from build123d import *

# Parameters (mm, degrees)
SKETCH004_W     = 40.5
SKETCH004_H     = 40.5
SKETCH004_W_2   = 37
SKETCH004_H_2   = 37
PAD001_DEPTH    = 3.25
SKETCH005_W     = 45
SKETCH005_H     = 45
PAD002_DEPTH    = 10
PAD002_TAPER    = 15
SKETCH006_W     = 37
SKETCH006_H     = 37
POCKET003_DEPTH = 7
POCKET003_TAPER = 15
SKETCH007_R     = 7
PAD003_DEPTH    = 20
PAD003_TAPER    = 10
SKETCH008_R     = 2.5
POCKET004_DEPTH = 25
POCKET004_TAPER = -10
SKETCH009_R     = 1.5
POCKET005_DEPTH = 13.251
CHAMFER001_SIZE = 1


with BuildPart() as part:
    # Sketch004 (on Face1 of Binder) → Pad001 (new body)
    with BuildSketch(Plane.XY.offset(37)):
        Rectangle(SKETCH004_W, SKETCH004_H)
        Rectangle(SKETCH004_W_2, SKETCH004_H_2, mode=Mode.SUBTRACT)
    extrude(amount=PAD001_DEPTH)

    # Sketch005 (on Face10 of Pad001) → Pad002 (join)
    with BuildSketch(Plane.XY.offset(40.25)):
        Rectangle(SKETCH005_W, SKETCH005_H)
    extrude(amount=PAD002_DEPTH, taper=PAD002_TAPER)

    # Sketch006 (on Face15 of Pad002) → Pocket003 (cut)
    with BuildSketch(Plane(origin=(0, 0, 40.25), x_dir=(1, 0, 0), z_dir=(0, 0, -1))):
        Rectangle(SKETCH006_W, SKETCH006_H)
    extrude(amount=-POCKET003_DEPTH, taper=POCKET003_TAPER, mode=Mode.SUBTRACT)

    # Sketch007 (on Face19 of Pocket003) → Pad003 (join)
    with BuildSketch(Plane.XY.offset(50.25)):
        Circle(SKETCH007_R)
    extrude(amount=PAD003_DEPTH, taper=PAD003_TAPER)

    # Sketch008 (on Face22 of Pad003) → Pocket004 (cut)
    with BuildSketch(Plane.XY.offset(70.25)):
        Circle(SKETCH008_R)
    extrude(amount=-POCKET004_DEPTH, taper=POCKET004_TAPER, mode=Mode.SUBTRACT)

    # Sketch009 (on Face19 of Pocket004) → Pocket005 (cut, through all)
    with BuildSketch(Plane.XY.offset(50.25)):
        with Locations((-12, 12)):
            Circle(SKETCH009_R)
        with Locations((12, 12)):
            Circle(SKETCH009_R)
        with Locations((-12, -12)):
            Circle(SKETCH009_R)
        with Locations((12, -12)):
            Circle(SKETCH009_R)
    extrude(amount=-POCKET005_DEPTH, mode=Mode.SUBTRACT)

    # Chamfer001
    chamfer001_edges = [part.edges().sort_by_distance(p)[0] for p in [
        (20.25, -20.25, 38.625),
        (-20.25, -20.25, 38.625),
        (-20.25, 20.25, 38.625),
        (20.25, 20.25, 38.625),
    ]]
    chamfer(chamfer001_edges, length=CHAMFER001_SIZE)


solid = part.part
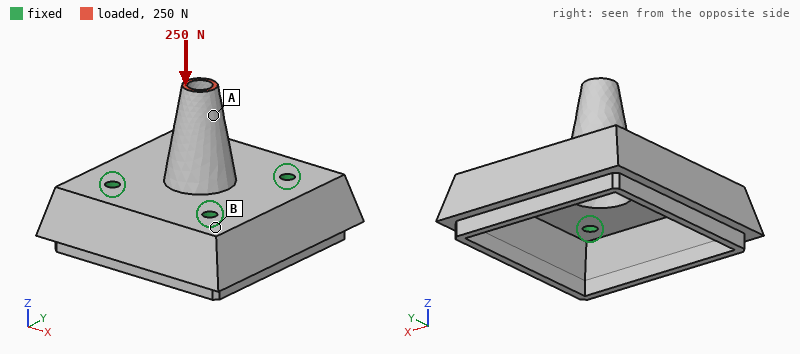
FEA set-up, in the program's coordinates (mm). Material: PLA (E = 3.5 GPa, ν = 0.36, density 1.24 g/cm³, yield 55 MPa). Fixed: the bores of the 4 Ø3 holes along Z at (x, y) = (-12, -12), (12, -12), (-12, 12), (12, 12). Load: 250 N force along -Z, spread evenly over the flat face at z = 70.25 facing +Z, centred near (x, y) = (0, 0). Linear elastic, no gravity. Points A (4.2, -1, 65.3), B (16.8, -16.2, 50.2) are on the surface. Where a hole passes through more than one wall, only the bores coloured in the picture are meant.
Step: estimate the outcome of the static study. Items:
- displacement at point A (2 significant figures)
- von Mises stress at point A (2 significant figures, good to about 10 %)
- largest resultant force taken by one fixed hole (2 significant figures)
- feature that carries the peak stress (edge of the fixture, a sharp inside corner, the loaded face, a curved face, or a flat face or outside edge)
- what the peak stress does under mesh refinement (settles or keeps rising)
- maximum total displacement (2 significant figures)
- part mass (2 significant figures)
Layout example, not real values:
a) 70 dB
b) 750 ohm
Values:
a) 0.13 mm
b) 11 MPa
c) 66 N
d) edge of the fixture
e) keeps rising
f) 0.16 mm
g) 13 g
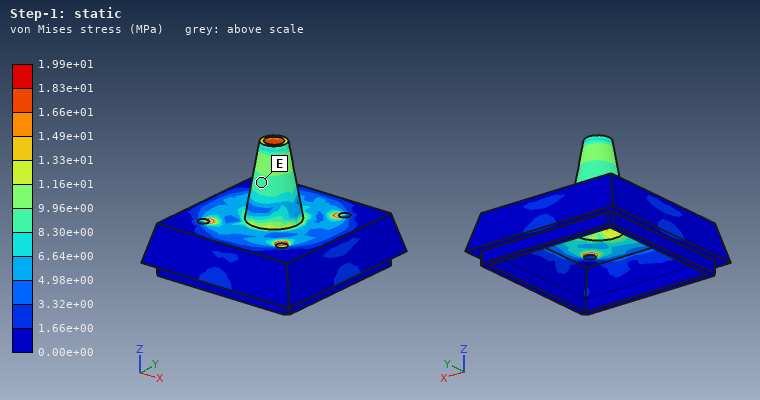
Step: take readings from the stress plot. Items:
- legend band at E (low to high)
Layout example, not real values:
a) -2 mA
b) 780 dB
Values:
a) 8.30e+00 to 9.96e+00 MPa
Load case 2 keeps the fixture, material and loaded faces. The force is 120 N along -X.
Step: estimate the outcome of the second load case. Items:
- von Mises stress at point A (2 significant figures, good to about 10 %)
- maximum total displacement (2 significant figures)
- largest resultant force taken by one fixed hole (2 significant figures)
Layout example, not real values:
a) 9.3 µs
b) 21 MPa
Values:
a) 15 MPa
b) 0.64 mm
c) 72 N
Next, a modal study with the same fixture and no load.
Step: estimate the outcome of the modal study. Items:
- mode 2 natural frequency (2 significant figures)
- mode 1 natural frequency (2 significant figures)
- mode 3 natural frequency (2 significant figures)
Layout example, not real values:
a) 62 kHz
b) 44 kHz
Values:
a) 4500 Hz
b) 4500 Hz
c) 4700 Hz
